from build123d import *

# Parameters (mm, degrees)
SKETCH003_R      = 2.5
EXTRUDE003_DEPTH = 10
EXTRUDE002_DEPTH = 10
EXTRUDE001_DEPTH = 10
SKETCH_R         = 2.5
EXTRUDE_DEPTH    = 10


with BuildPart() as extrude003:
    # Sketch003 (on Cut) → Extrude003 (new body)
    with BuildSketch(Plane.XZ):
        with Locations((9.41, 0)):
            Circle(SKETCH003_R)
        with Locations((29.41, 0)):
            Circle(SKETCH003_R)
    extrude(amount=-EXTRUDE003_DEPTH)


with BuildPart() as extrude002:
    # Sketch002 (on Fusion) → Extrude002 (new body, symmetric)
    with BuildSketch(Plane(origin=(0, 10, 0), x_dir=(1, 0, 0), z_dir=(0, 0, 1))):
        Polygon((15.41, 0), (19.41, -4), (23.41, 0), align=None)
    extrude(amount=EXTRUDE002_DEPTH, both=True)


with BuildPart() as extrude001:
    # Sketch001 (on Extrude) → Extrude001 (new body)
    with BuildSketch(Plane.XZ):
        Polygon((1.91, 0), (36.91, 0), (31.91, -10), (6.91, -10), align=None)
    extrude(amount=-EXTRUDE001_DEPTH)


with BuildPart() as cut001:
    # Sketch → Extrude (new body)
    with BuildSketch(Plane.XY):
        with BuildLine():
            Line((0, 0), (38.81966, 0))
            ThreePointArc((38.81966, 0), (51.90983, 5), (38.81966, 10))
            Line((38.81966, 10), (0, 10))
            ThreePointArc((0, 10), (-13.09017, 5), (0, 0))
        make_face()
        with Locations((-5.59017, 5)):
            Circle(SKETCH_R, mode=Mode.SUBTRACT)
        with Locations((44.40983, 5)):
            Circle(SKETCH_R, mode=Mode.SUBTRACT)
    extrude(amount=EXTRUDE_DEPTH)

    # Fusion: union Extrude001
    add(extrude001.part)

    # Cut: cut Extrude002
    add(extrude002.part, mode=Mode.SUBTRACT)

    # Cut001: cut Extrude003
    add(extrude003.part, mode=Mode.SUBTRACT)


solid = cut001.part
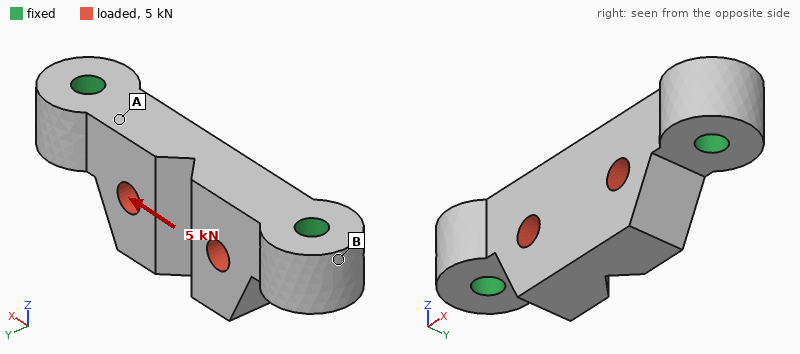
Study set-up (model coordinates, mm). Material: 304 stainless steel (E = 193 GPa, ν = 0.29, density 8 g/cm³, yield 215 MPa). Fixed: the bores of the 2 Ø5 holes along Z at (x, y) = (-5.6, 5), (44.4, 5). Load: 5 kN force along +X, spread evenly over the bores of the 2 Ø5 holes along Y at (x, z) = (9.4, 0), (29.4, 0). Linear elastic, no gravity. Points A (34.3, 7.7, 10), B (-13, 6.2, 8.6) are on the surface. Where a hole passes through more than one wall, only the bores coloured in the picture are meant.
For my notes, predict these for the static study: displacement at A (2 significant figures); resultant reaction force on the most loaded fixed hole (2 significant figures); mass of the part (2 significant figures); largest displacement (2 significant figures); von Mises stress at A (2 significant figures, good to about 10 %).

0.98 µm
2.6 kN
72 g
3.0 µm
12 MPa
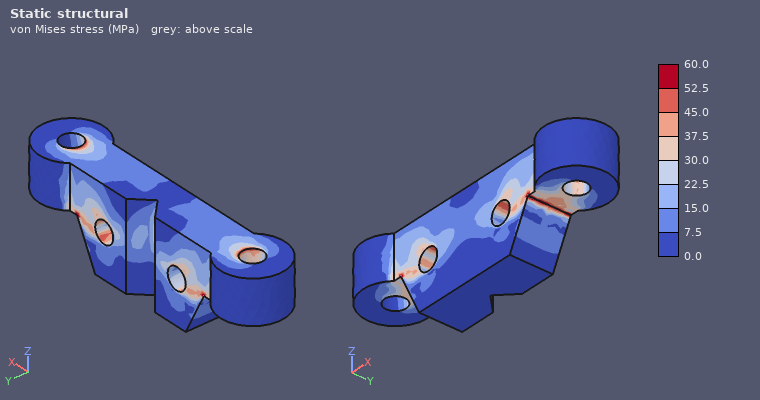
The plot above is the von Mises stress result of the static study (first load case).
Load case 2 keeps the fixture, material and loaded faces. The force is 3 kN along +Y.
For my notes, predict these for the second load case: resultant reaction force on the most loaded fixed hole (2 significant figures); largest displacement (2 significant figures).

1.5 kN
19 µm
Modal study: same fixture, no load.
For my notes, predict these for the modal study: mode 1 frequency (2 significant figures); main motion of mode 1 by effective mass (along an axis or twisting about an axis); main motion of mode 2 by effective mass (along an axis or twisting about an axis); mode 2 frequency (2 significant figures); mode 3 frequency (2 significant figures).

11 kHz
along Y
along Z
19 kHz
20 kHz
